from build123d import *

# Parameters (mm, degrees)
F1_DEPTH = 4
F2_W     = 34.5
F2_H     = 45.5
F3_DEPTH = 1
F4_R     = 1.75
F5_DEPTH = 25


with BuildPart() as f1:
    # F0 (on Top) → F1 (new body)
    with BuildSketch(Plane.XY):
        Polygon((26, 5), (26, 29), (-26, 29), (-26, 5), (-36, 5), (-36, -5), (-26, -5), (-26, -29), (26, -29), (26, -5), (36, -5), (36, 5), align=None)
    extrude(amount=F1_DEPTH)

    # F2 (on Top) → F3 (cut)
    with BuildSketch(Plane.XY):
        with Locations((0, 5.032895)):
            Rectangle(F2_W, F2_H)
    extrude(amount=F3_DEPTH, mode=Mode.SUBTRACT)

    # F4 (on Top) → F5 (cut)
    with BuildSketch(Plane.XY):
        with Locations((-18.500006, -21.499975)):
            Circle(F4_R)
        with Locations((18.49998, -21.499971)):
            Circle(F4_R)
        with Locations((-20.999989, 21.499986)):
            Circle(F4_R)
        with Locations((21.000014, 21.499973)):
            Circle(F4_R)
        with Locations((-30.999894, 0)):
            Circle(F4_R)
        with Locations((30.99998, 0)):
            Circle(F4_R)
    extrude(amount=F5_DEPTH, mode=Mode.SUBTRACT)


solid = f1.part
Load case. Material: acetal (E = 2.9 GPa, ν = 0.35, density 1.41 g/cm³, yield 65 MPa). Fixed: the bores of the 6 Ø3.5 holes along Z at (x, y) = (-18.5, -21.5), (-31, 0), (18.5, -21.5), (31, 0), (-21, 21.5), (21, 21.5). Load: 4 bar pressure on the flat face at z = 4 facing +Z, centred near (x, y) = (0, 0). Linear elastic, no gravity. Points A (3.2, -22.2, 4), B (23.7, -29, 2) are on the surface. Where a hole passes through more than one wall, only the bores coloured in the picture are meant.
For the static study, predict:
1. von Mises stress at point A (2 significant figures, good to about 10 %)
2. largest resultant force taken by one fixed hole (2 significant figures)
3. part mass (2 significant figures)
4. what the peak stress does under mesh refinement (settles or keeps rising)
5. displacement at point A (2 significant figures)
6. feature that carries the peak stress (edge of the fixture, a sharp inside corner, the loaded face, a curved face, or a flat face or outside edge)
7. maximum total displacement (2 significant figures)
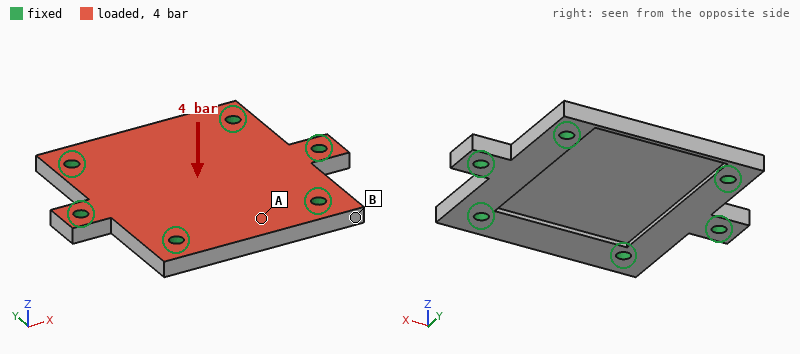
12 MPa
260 N
16 g
keeps rising
0.20 mm
edge of the fixture
0.66 mm
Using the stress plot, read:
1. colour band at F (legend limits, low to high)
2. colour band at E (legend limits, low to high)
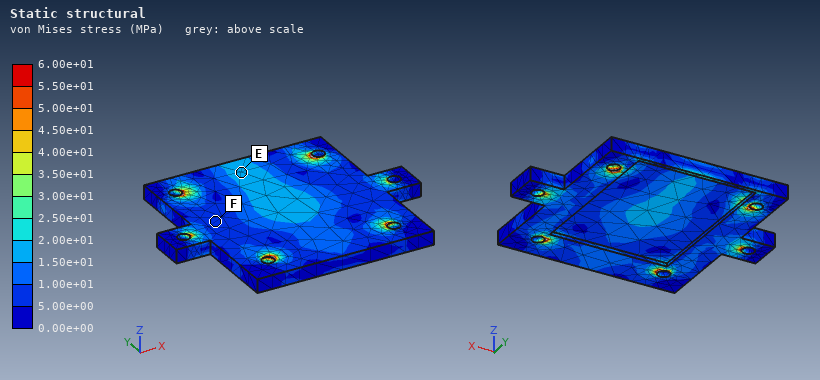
5.00e+00 to 1.00e+01 MPa
1.50e+01 to 2.00e+01 MPa
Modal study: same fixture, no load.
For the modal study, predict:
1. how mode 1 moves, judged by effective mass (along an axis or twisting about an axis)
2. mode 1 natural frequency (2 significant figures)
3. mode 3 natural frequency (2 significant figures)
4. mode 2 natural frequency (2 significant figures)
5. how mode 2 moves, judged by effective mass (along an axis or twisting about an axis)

along Z
2400 Hz
4300 Hz
3300 Hz
twisting about X
